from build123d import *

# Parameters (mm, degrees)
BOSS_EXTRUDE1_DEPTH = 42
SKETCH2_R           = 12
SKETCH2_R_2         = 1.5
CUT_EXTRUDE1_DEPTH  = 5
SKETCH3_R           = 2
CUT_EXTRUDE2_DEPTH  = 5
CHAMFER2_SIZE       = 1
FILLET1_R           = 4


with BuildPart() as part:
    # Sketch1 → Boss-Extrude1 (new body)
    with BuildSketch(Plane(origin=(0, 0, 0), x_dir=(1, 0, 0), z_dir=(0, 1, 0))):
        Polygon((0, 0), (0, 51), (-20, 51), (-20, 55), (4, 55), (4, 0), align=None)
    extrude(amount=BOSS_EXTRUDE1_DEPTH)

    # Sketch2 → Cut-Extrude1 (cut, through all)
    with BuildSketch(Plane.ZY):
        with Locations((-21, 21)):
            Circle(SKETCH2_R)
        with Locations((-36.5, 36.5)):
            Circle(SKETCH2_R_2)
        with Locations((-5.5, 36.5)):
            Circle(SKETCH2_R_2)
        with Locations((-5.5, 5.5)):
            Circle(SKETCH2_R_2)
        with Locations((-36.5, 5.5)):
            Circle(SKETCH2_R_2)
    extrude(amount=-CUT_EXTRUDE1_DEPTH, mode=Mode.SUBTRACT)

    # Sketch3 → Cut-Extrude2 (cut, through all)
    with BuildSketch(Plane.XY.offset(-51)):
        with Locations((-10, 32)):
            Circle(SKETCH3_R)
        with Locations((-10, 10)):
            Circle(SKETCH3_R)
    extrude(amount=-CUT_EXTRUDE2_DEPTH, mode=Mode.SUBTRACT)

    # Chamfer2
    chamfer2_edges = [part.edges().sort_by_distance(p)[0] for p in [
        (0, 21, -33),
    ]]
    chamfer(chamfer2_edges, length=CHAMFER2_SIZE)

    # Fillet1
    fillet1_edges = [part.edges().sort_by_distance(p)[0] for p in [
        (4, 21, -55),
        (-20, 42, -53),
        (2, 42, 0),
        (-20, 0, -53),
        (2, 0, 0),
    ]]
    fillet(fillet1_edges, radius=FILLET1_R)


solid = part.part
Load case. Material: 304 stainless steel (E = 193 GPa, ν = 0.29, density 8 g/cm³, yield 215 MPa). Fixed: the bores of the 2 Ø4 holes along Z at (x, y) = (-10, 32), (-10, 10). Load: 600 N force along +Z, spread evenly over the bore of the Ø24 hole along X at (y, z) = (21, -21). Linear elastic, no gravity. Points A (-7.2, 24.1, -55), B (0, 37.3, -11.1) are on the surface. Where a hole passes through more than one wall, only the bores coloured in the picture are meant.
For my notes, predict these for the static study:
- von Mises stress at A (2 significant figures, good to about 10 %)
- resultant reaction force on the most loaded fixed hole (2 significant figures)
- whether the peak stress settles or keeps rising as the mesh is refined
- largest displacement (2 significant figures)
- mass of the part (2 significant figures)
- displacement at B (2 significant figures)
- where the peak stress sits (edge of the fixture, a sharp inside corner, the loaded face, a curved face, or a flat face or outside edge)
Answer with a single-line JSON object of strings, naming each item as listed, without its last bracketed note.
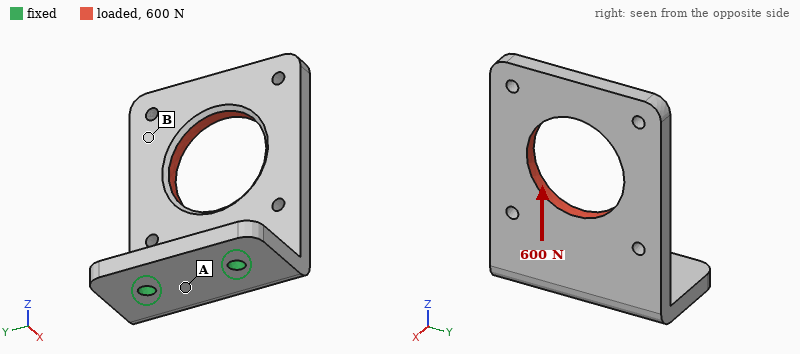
{"von Mises stress at A": "29 MPa", "resultant reaction force on the most loaded fixed hole": "300 N", "whether the peak stress settles or keeps rising as the mesh is refined": "keeps rising", "largest displacement": "70 µm", "mass of the part": "83 g", "displacement at B": "53 µm", "where the peak stress sits": "edge of the fixture"}
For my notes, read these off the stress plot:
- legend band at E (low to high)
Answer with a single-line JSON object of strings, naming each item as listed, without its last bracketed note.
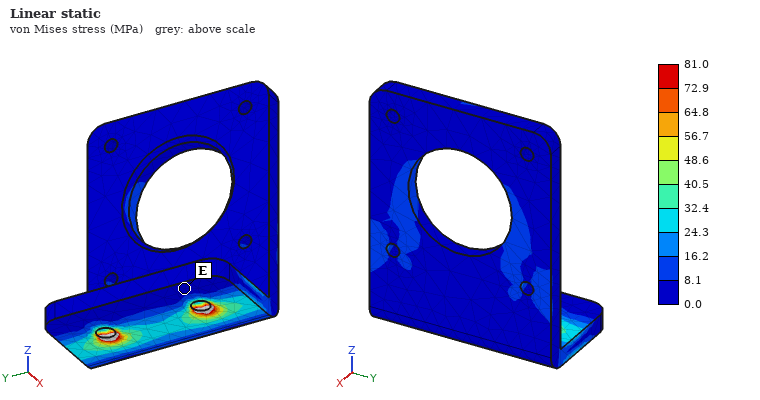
{"legend band at E": "0.0 to 8.1 MPa"}
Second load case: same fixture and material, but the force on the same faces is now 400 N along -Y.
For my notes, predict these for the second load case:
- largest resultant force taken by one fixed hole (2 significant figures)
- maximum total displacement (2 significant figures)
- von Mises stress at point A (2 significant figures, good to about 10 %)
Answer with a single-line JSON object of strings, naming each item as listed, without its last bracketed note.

{"largest resultant force taken by one fixed hole": "550 N", "maximum total displacement": "44 µm", "von Mises stress at point A": "17 MPa"}
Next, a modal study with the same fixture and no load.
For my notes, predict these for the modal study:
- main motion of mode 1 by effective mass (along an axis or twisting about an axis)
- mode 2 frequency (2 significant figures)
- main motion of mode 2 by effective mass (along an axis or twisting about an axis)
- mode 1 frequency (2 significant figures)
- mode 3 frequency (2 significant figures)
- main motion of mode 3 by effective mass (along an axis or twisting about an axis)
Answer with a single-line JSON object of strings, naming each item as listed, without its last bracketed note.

{"main motion of mode 1 by effective mass": "along X", "mode 2 frequency": "2400 Hz", "main motion of mode 2 by effective mass": "along Y", "mode 1 frequency": "910 Hz", "mode 3 frequency": "3100 Hz", "main motion of mode 3 by effective mass": "along Y"}
